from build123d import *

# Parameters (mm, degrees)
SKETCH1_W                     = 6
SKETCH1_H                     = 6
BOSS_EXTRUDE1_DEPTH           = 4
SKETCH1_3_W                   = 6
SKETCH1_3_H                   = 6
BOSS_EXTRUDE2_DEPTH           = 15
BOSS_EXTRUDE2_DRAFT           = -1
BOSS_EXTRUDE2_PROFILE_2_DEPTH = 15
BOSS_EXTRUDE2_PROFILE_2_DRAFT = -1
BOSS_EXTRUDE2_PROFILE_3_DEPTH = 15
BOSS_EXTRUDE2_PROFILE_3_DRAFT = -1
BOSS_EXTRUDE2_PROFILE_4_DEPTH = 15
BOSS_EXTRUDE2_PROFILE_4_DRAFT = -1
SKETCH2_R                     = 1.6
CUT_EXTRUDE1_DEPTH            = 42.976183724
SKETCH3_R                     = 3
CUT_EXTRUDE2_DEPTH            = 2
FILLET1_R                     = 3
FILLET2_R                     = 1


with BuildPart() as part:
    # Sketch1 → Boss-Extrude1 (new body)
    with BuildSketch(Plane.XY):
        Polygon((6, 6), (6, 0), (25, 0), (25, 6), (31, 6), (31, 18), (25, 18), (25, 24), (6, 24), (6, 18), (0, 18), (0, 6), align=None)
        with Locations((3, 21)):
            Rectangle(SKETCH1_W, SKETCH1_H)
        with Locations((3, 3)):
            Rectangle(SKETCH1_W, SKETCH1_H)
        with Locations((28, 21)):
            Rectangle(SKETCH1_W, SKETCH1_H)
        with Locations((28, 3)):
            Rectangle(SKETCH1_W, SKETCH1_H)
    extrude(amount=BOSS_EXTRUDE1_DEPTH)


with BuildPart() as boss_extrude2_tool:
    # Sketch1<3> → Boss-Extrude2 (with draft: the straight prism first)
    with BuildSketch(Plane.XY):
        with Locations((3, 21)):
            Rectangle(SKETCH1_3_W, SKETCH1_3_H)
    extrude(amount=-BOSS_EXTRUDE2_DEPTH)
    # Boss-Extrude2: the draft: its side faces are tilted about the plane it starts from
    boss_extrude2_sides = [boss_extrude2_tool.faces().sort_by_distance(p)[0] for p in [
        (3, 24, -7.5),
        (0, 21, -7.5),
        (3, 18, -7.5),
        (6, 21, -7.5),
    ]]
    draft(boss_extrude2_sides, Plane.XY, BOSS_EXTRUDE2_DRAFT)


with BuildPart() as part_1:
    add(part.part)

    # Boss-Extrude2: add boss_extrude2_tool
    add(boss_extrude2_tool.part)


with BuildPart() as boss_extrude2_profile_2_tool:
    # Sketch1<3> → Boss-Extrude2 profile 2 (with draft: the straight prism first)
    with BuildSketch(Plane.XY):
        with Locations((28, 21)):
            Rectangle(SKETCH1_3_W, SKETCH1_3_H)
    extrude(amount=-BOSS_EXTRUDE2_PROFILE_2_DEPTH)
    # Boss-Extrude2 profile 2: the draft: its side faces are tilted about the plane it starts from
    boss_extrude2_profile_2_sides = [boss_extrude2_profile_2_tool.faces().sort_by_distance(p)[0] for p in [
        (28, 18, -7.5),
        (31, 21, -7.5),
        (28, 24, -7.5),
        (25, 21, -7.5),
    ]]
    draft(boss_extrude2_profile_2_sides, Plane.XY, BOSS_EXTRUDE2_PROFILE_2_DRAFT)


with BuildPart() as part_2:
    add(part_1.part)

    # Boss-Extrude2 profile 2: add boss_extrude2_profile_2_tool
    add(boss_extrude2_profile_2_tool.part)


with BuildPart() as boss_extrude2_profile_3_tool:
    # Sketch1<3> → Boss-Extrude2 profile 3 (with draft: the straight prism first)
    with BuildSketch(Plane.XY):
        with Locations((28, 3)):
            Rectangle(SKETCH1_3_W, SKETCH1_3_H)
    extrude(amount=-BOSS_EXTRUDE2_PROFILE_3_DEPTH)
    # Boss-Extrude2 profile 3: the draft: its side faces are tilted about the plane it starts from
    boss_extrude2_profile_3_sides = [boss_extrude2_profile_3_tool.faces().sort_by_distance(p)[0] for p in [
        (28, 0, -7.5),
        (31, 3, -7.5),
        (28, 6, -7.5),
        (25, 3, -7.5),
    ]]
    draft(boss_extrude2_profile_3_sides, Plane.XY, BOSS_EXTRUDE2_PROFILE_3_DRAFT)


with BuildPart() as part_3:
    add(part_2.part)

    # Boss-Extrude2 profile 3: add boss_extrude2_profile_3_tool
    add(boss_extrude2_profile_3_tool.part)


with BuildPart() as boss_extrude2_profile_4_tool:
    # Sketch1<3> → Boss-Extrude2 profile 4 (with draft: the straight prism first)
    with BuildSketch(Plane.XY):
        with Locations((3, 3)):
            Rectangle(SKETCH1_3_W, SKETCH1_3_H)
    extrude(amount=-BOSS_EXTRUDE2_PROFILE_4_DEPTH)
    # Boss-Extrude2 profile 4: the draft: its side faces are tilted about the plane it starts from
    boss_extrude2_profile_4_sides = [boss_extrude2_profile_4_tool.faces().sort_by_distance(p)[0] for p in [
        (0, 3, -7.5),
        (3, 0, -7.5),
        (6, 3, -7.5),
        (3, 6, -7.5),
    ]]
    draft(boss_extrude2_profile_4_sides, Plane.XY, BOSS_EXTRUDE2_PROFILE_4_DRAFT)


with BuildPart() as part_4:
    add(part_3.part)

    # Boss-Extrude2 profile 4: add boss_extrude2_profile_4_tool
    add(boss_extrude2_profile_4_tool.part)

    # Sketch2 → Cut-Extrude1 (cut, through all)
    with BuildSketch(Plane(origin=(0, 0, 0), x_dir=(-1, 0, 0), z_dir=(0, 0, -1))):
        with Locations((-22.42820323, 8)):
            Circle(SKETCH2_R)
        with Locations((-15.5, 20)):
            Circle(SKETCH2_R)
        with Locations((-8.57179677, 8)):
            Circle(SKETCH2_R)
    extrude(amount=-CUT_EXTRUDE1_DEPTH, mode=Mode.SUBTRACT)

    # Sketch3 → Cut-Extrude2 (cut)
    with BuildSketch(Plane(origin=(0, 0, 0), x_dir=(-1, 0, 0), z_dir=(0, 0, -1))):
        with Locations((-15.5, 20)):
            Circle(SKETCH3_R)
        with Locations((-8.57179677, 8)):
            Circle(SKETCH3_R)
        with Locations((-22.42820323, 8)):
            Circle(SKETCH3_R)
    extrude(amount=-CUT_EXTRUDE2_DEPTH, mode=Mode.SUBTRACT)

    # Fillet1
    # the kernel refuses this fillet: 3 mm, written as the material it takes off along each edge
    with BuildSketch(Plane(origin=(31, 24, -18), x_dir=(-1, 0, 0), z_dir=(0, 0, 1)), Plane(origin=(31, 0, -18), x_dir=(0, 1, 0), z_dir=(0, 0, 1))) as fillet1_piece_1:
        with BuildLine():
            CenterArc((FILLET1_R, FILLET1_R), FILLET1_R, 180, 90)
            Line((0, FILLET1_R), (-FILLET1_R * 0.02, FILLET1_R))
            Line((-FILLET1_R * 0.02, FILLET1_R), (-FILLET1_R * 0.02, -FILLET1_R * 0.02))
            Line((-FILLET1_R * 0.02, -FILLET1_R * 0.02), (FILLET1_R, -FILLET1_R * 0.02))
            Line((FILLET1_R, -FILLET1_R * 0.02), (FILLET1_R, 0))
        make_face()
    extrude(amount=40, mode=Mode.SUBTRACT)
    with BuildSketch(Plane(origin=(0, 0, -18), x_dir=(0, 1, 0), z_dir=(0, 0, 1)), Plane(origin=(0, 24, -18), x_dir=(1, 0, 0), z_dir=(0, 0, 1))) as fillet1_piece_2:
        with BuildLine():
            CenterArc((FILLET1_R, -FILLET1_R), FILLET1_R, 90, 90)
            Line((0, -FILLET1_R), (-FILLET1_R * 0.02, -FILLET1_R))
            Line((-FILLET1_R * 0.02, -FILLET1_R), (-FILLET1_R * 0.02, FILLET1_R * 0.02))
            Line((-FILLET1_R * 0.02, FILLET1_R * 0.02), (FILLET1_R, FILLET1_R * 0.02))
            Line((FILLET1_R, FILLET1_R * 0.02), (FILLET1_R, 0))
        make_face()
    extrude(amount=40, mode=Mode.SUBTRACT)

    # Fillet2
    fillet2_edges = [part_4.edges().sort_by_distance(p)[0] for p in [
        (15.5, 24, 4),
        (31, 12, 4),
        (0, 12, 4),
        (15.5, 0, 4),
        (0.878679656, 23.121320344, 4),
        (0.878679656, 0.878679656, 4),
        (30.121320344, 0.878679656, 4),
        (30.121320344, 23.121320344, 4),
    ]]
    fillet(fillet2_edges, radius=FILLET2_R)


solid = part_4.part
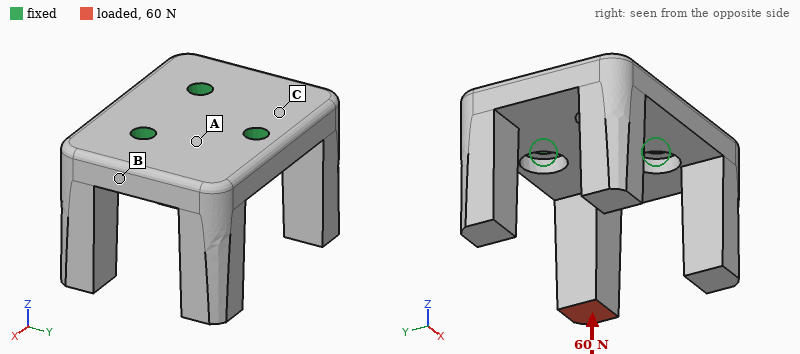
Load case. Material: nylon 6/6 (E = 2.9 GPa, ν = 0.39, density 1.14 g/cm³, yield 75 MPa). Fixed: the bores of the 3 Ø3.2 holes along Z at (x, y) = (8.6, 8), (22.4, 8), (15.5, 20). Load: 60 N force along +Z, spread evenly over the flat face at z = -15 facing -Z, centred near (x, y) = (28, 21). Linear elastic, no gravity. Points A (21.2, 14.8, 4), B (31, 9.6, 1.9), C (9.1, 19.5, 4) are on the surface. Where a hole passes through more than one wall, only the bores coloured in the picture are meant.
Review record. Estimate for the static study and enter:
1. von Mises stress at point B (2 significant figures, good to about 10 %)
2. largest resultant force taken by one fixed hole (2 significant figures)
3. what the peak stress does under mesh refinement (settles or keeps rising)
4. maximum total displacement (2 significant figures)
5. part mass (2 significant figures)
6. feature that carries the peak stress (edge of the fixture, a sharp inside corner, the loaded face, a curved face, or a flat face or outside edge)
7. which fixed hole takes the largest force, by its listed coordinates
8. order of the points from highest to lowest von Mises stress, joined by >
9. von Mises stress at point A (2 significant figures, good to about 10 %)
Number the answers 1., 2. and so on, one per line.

1. 5.0 MPa
2. 58 N
3. keeps rising
4. 0.44 mm
5. 5.2 g
6. edge of the fixture
7. (15.5, 20)
8. A > B > C
9. 8.4 MPa
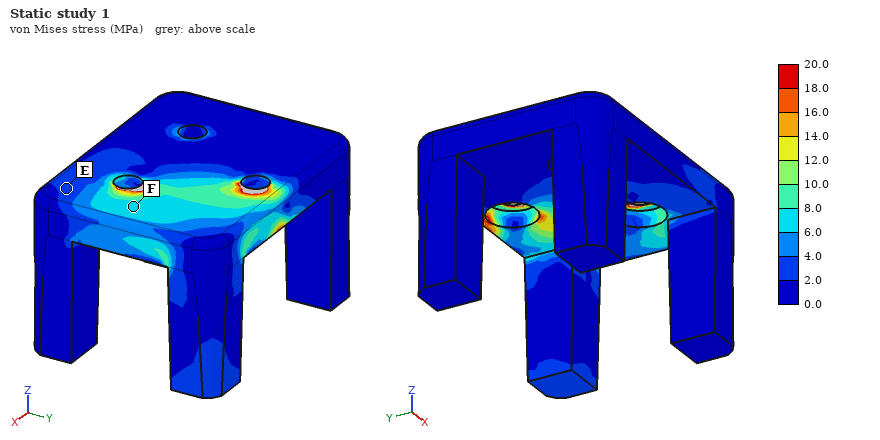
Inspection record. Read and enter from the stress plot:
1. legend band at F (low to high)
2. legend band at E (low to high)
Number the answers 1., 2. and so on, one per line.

1. 6.0 to 8.0 MPa
2. 2.0 to 4.0 MPa
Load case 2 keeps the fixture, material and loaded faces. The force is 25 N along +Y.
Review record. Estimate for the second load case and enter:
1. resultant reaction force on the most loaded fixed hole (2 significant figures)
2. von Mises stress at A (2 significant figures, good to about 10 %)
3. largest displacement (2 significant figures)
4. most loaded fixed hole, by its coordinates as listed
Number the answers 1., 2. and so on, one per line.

1. 41 N
2. 4.4 MPa
3. 0.45 mm
4. (15.5, 20)
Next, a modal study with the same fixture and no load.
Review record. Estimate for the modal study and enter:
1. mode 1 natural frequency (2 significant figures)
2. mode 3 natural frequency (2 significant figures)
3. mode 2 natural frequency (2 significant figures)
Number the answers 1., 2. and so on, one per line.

1. 2000 Hz
2. 2400 Hz
3. 2100 Hz
